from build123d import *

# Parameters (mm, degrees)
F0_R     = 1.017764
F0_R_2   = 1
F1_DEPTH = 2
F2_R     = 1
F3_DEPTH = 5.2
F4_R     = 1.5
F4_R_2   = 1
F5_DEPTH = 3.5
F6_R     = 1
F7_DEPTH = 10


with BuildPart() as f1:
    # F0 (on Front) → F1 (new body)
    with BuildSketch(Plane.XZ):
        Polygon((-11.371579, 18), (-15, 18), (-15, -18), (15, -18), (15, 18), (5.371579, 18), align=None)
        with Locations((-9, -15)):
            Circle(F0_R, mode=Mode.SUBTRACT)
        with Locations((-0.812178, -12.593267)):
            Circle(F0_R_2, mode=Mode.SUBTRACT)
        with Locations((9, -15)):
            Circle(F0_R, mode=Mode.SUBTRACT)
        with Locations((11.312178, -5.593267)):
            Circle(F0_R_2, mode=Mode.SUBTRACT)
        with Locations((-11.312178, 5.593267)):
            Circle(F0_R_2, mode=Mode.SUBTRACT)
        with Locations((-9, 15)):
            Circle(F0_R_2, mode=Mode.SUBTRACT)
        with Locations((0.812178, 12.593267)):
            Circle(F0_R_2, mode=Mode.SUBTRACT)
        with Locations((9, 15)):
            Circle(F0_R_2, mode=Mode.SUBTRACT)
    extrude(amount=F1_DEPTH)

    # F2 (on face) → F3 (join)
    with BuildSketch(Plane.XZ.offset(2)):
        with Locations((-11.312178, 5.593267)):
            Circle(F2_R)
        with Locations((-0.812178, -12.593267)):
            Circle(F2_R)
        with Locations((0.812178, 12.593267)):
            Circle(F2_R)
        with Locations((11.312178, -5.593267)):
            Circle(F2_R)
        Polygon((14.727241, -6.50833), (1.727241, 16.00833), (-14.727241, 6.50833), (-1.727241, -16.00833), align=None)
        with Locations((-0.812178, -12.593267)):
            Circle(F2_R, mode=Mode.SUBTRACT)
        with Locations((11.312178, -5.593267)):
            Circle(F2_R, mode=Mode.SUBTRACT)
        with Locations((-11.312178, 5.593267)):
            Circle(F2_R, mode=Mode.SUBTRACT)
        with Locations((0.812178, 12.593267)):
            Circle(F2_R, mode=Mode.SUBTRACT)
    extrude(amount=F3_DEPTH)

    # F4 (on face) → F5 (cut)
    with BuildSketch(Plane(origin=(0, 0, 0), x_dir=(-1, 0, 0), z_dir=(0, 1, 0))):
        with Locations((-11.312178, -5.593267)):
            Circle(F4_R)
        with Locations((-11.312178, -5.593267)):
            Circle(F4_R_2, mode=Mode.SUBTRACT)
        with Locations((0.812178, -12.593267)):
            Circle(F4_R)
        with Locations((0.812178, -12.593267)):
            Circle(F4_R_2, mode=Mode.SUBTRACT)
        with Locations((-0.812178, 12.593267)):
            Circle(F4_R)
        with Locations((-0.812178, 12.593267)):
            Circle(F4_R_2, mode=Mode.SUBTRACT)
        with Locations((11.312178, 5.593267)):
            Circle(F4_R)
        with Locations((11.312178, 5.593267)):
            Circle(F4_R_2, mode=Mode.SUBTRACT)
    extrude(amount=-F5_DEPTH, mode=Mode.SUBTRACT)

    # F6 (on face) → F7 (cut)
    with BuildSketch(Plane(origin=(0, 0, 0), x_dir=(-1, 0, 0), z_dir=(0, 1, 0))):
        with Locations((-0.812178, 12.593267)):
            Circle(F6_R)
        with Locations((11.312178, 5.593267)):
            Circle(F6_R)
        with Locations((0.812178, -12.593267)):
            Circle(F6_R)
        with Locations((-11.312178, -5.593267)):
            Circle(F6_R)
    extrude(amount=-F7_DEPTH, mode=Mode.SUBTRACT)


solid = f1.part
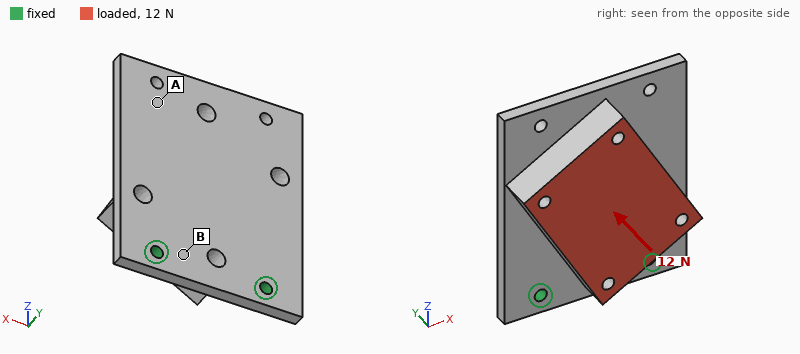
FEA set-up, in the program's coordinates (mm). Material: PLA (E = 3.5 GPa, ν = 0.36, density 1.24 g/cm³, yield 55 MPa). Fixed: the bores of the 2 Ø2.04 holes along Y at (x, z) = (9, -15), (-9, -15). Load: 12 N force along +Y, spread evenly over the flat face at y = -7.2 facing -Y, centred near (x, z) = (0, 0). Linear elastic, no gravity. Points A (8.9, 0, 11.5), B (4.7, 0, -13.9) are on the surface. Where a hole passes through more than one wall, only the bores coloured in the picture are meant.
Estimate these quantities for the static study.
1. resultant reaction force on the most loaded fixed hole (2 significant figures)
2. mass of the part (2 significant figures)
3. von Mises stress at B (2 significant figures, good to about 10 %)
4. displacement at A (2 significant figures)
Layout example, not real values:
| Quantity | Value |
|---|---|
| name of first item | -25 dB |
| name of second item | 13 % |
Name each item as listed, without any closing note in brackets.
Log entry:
| Quantity | Value |
|---|---|
| resultant reaction force on the most loaded fixed hole | 6.3 N |
| mass of the part | 5.7 g |
| von Mises stress at B | 5.2 MPa |
| displacement at A | 0.28 mm |
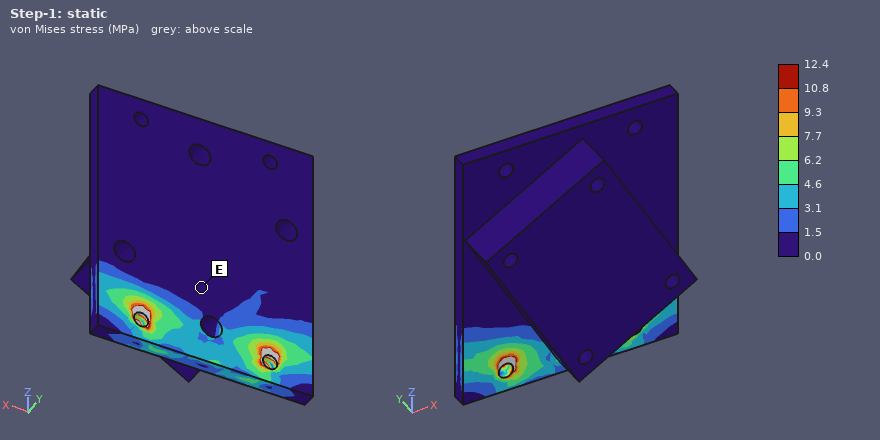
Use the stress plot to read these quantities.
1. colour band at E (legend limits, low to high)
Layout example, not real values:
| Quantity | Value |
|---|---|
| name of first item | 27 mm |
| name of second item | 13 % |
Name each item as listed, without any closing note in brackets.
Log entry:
| Quantity | Value |
|---|---|
| colour band at E | 0.0 to 1.5 MPa |
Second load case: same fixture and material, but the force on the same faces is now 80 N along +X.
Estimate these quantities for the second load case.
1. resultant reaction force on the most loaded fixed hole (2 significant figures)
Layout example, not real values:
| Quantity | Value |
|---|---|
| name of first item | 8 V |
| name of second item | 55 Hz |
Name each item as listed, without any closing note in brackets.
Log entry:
| Quantity | Value |
|---|---|
| resultant reaction force on the most loaded fixed hole | 80 N |
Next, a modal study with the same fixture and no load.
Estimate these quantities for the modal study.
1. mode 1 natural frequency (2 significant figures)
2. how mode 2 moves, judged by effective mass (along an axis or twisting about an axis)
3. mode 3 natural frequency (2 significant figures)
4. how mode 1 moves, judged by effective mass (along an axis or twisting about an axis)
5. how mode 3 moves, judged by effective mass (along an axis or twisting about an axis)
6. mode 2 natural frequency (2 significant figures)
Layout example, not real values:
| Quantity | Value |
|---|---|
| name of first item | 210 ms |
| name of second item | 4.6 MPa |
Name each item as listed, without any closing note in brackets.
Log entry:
| Quantity | Value |
|---|---|
| mode 1 natural frequency | 490 Hz |
| how mode 2 moves, judged by effective mass | twisting about Z |
| mode 3 natural frequency | 3300 Hz |
| how mode 1 moves, judged by effective mass | along Y |
| how mode 3 moves, judged by effective mass | along X |
| mode 2 natural frequency | 2600 Hz |
